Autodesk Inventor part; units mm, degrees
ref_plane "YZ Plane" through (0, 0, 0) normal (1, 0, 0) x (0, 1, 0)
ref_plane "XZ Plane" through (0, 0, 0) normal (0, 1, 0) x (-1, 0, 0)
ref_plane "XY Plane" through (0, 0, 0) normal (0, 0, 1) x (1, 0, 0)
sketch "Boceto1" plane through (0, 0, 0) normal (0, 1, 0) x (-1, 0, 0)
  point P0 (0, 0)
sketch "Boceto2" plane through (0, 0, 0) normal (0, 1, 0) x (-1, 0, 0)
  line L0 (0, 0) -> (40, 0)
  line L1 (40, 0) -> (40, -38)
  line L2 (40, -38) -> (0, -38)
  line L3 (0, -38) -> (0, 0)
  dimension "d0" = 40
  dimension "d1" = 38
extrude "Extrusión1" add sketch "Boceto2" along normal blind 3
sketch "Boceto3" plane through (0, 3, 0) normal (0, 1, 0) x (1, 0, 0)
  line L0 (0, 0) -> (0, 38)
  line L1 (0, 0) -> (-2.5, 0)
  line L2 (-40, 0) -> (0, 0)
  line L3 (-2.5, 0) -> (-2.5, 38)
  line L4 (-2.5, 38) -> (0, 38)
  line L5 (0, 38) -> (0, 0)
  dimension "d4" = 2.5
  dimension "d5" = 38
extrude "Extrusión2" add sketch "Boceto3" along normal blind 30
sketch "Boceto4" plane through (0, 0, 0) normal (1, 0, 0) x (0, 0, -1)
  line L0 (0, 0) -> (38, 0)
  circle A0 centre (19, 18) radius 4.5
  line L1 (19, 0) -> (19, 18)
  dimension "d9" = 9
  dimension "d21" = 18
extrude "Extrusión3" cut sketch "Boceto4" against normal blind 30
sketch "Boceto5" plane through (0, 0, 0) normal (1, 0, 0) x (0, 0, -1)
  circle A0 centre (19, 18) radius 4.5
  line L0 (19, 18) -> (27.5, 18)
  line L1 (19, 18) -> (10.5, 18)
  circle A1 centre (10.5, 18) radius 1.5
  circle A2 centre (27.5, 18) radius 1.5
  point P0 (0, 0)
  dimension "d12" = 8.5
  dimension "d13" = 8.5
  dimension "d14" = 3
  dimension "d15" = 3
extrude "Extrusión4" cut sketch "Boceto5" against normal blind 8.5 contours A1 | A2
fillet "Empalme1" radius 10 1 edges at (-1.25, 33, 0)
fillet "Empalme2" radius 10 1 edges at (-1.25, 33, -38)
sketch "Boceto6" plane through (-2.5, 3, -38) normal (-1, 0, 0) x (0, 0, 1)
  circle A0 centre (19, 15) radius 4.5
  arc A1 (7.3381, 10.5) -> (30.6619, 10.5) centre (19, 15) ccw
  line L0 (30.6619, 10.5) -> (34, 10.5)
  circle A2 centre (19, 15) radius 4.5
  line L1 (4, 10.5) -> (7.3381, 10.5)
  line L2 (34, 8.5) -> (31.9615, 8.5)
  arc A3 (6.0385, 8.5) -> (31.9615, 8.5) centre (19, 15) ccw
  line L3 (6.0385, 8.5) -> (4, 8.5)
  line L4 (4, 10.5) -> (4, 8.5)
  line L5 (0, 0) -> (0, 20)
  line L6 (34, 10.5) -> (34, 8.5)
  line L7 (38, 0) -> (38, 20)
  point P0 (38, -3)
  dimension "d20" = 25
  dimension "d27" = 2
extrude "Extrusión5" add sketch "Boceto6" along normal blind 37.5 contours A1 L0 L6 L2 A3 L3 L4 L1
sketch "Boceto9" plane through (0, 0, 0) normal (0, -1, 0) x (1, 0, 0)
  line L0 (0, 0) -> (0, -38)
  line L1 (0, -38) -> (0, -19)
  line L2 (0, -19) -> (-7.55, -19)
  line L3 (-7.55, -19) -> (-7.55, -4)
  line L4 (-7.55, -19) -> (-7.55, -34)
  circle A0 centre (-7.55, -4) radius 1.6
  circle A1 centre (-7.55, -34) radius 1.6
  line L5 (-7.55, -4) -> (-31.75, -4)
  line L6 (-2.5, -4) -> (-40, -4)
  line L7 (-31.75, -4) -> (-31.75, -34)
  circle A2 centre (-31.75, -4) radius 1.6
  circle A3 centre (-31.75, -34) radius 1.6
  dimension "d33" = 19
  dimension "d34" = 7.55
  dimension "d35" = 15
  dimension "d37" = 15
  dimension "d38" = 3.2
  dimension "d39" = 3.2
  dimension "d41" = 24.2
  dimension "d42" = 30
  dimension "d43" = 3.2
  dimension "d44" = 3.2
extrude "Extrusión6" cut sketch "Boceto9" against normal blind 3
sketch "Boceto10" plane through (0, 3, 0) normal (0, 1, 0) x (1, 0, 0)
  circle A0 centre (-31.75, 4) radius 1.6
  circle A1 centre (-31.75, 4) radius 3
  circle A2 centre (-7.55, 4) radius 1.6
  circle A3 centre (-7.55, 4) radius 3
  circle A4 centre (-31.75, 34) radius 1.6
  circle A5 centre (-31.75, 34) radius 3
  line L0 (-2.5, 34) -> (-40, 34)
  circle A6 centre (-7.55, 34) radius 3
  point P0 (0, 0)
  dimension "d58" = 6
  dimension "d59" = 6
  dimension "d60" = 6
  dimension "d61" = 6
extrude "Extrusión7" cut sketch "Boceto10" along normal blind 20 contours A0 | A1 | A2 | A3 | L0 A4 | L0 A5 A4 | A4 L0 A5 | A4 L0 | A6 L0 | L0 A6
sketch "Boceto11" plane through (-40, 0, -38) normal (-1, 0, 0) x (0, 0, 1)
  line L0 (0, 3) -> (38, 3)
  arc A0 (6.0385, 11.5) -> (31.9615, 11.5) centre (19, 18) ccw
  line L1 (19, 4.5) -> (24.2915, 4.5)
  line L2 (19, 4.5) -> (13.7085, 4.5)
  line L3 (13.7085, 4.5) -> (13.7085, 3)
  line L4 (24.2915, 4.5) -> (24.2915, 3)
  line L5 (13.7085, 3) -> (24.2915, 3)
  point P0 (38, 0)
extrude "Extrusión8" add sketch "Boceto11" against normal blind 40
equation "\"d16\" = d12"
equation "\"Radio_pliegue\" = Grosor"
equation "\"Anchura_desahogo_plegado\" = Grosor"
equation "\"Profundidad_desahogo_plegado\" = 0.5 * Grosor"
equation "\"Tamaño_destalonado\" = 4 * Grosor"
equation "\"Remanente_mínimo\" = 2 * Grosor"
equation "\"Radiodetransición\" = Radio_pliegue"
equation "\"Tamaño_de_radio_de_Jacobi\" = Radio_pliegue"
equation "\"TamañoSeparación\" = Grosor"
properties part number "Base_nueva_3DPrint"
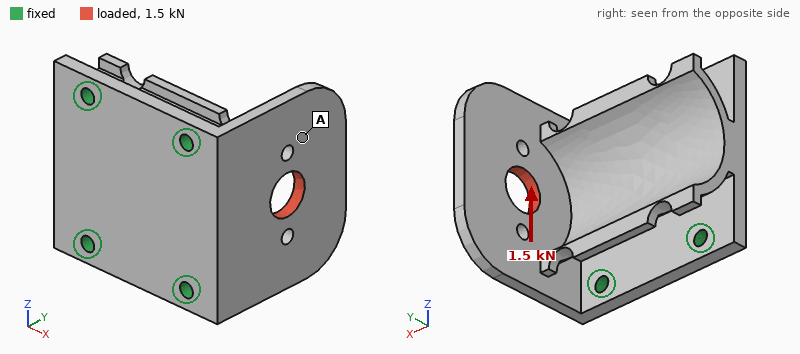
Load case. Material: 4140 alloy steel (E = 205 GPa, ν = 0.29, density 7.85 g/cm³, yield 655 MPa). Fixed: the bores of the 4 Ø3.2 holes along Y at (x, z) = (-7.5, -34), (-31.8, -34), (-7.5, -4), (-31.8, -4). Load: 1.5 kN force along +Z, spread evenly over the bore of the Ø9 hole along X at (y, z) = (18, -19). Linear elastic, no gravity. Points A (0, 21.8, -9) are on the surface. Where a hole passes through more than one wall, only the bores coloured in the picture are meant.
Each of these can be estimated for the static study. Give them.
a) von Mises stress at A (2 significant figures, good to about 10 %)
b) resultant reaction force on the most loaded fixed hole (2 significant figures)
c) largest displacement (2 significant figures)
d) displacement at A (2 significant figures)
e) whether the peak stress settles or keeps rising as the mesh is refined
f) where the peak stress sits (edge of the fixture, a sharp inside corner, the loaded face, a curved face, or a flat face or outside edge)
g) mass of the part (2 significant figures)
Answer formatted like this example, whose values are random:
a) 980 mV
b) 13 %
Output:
a) 18 MPa
b) 1.1 kN
c) 22 µm
d) 16 µm
e) keeps rising
f) edge of the fixture
g) 78 g
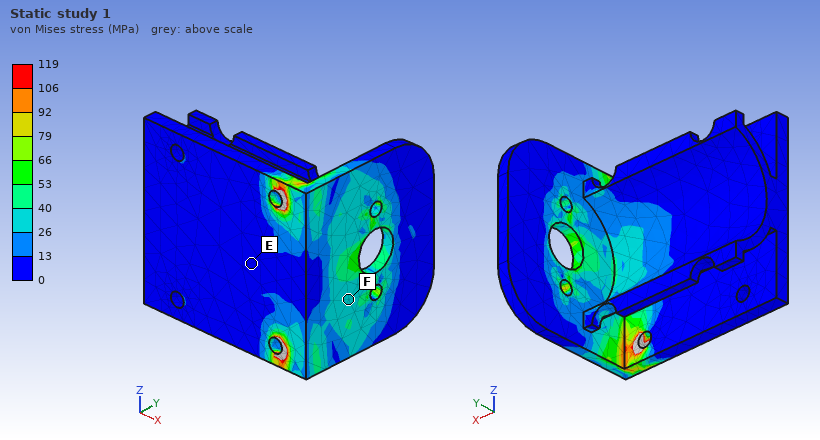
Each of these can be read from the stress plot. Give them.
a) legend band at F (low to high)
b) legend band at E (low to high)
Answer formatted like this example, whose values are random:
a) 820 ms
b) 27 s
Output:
a) 26 to 40 MPa
b) 0 to 13 MPa
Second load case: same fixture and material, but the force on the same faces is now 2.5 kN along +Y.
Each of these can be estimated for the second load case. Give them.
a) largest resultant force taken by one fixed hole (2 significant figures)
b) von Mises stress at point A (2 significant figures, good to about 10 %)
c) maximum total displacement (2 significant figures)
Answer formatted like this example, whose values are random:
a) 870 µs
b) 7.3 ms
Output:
a) 1.4 kN
b) 28 MPa
c) 21 µm
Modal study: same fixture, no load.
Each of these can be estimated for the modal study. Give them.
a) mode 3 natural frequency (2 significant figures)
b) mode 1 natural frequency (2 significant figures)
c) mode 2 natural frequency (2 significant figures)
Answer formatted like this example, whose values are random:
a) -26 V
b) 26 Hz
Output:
a) 8900 Hz
b) 3500 Hz
c) 7300 Hz
